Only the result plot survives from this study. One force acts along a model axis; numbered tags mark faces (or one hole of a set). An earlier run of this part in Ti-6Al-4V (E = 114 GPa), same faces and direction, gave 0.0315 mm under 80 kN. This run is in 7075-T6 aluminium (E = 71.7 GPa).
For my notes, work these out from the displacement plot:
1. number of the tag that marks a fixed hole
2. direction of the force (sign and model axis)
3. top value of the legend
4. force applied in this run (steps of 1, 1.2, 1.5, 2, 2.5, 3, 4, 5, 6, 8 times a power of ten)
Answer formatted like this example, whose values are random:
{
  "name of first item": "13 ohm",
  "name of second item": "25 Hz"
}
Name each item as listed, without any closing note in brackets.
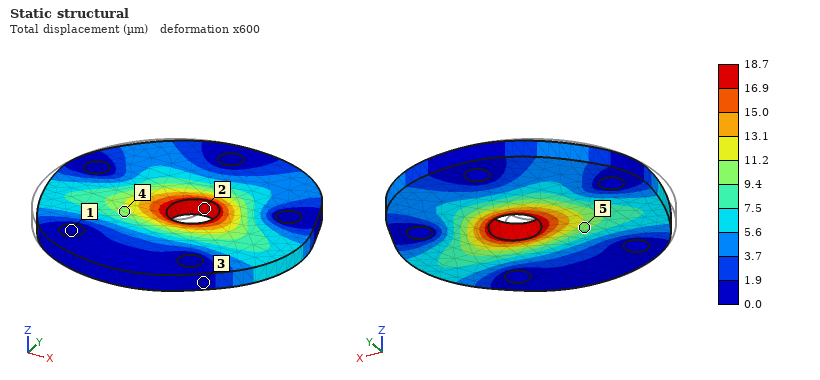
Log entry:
{
  "number of the tag that marks a fixed hole": "1",
  "direction of the force": "+X",
  "top value of the legend": "18.7 µm",
  "force applied in this run": "30 kN"
}
